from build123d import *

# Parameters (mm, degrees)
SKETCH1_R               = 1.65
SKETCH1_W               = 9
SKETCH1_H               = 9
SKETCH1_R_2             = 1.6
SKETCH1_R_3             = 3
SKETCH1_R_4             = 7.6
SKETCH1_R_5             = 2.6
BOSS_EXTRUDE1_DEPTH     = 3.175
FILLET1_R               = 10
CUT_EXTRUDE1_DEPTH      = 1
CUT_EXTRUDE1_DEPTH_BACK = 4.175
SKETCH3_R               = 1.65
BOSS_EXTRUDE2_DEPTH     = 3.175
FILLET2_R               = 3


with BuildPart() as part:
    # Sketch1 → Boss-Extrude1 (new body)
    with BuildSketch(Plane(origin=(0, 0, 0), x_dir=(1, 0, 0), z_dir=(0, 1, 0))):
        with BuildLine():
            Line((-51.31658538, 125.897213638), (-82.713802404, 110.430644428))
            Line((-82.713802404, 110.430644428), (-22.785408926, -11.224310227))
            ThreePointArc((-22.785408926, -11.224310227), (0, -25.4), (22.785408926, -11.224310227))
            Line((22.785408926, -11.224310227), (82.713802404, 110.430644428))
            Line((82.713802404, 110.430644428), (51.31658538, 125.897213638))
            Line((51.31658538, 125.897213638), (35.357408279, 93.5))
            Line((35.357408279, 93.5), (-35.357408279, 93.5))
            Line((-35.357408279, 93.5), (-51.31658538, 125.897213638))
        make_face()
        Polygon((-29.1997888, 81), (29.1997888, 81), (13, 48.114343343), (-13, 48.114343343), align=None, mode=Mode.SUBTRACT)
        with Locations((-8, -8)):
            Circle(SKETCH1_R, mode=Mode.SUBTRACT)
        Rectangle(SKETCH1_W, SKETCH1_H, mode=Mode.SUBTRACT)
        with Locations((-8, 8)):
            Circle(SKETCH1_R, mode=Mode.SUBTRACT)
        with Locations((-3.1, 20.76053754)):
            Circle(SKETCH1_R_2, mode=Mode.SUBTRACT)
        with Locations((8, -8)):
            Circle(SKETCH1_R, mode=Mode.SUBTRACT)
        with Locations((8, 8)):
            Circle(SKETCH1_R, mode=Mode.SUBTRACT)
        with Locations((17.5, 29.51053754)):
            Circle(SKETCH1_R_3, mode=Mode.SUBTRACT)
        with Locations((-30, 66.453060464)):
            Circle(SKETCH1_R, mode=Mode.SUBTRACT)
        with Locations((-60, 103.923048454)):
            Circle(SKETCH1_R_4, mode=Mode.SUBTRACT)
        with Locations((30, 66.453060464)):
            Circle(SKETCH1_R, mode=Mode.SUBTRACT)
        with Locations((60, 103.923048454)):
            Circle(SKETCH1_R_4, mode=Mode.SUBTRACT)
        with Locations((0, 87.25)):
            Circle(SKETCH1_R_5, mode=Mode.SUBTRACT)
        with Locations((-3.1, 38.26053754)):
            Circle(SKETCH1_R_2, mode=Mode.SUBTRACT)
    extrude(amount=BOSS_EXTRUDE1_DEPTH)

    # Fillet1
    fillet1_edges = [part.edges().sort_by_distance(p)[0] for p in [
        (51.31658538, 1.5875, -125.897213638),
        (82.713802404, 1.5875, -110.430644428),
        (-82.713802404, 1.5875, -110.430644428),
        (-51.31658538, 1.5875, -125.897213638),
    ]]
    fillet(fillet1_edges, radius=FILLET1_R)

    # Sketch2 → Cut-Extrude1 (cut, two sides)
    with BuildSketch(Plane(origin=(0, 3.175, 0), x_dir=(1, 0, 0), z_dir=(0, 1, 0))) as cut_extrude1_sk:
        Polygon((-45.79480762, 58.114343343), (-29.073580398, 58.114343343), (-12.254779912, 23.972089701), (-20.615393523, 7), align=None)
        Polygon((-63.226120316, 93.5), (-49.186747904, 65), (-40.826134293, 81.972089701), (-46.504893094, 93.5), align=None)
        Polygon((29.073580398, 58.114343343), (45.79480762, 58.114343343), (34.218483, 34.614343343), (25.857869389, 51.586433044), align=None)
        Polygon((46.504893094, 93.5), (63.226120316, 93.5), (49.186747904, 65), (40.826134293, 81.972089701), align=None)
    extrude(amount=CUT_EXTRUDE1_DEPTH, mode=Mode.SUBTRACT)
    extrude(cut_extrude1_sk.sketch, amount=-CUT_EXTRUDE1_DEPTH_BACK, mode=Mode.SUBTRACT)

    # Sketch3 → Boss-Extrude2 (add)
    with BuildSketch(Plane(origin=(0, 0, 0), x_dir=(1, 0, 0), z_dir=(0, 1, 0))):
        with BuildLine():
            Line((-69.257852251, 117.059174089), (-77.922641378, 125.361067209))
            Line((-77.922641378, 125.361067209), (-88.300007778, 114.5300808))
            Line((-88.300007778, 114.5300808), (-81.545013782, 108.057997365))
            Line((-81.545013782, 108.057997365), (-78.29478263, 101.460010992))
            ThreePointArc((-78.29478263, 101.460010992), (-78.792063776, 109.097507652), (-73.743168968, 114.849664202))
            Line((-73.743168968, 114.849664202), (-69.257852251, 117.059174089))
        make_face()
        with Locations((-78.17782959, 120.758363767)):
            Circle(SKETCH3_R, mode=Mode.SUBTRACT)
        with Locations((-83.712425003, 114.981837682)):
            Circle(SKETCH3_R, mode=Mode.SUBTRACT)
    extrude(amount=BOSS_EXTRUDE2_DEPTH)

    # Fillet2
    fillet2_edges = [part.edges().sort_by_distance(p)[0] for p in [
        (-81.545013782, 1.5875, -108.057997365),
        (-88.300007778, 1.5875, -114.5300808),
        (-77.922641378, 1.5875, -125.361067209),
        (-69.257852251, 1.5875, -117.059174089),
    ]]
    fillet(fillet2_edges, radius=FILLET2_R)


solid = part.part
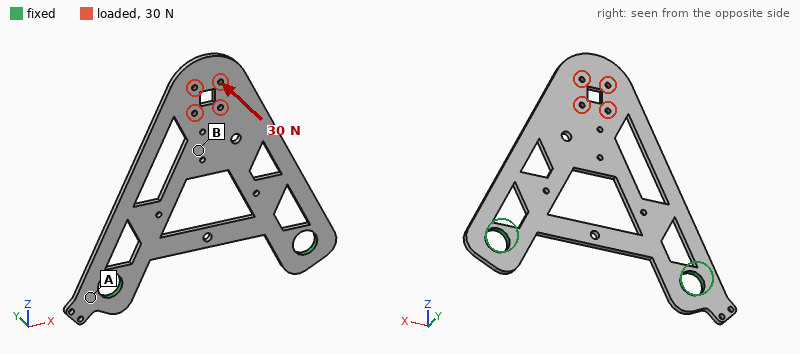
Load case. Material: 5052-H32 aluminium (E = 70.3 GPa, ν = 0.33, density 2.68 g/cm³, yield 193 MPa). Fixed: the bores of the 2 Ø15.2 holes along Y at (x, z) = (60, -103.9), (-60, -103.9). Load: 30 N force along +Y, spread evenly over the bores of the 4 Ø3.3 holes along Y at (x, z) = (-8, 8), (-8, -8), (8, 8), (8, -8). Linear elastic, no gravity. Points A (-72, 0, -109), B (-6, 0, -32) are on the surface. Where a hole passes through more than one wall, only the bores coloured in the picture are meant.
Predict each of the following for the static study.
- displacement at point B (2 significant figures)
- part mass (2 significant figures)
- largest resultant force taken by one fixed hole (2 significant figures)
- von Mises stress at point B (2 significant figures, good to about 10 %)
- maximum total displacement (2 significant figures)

0.74 mm
77 g
15 N
10 MPa
1.7 mm
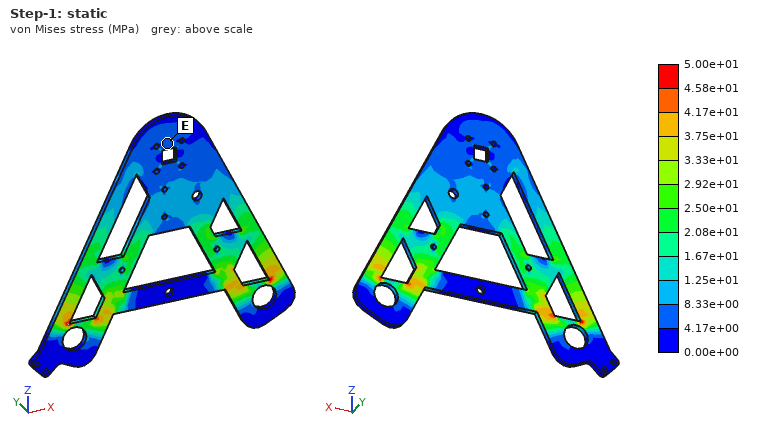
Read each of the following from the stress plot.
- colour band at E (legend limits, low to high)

4.17e+00 to 8.33e+00 MPa
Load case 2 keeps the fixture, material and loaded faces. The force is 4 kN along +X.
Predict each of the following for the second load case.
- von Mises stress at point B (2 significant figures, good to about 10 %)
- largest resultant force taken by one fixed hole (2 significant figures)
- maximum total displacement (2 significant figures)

42 MPa
3.8 kN
0.19 mm
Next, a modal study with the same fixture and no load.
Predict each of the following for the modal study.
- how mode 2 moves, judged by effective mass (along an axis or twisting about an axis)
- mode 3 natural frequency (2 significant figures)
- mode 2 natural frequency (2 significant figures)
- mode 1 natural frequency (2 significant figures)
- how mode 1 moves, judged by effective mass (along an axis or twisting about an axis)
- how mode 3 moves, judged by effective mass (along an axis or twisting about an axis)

twisting about Z
870 Hz
740 Hz
160 Hz
along Y
along Y
